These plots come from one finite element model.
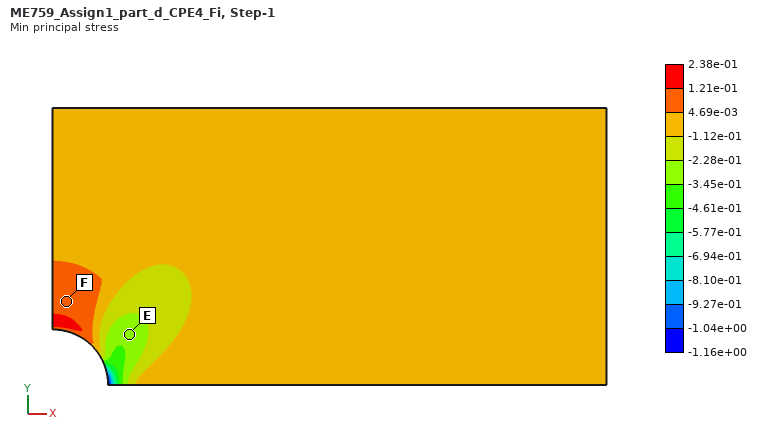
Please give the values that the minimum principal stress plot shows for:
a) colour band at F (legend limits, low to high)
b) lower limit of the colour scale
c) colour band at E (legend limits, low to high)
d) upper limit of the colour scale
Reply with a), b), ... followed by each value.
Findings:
a) 4.69e-03 to 1.21e-01
b) -1.16e+00
c) -3.45e-01 to -2.28e-01
d) 2.38e-01
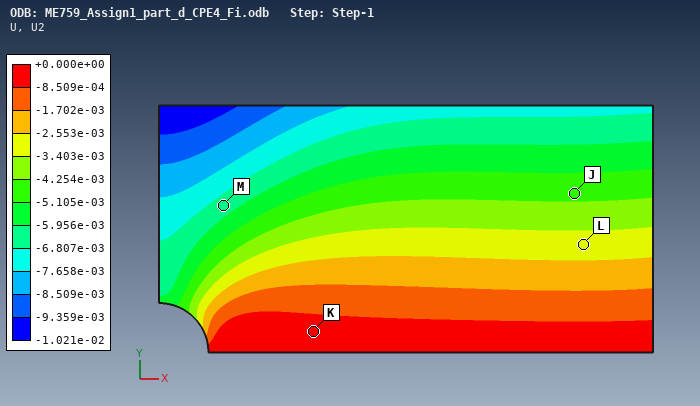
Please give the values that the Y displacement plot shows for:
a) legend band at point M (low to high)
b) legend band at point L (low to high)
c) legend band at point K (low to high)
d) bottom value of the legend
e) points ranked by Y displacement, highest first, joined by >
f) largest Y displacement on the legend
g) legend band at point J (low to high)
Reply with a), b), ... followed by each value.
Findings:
a) -6.807e-03 to -5.956e-03
b) -3.403e-03 to -2.553e-03
c) -8.509e-04 to +0.000e+00
d) -1.021e-02
e) K > L > J > M
f) +0.000e+00
g) -5.105e-03 to -4.254e-03
